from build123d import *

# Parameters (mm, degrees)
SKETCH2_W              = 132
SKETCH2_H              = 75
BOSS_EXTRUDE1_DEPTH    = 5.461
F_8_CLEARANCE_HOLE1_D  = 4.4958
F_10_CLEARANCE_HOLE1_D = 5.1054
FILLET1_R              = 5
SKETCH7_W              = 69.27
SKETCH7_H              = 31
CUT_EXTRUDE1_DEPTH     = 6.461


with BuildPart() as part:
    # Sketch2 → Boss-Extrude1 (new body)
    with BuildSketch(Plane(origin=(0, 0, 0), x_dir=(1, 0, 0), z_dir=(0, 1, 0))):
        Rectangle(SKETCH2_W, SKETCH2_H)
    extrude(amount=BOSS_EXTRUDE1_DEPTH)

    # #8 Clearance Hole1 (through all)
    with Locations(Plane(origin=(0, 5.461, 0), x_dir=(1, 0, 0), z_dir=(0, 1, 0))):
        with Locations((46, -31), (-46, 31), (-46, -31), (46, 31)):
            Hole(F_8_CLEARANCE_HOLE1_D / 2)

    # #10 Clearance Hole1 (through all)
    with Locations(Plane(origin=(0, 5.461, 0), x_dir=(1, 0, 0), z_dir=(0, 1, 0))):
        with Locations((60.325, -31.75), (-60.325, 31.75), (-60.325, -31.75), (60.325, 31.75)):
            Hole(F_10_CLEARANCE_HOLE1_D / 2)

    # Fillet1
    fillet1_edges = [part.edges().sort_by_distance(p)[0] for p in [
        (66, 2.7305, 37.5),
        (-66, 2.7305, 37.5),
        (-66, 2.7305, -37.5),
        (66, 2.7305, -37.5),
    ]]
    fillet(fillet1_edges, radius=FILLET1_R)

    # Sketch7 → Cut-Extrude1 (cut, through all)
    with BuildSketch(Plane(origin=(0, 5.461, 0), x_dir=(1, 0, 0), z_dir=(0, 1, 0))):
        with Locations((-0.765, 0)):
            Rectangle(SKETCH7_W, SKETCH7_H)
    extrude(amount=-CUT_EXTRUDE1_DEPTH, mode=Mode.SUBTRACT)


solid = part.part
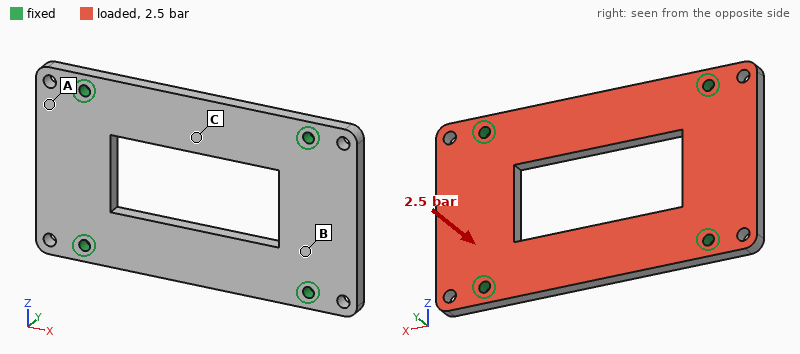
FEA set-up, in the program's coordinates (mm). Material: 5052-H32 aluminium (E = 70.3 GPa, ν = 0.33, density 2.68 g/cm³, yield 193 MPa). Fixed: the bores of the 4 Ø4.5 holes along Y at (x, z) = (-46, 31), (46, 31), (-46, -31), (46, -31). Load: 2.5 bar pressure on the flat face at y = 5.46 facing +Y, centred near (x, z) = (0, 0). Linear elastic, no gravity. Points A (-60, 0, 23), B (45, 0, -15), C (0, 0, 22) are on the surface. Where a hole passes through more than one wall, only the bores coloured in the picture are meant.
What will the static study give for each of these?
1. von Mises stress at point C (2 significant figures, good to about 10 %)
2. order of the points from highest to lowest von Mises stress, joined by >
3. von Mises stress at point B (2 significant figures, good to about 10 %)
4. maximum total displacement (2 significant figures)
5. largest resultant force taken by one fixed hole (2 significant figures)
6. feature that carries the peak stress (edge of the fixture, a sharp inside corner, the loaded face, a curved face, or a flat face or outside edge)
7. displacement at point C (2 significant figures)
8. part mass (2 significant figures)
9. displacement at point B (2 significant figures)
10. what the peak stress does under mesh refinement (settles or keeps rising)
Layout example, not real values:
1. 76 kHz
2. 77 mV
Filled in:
1. 17 MPa
2. C > B > A
3. 11 MPa
4. 58 µm
5. 480 N
6. edge of the fixture
7. 53 µm
8. 110 g
9. 12 µm
10. keeps rising
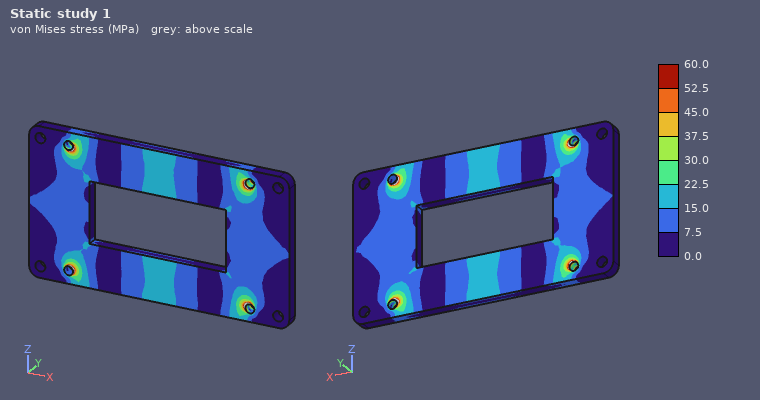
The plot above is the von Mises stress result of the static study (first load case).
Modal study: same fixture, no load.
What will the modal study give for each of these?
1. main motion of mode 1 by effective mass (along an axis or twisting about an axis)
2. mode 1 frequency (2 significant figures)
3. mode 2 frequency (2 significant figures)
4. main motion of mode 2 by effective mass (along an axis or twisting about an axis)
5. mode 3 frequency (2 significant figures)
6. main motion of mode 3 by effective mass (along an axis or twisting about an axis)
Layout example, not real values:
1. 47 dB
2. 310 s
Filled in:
1. along Y
2. 3200 Hz
3. 3400 Hz
4. twisting about X
5. 5600 Hz
6. along Y
